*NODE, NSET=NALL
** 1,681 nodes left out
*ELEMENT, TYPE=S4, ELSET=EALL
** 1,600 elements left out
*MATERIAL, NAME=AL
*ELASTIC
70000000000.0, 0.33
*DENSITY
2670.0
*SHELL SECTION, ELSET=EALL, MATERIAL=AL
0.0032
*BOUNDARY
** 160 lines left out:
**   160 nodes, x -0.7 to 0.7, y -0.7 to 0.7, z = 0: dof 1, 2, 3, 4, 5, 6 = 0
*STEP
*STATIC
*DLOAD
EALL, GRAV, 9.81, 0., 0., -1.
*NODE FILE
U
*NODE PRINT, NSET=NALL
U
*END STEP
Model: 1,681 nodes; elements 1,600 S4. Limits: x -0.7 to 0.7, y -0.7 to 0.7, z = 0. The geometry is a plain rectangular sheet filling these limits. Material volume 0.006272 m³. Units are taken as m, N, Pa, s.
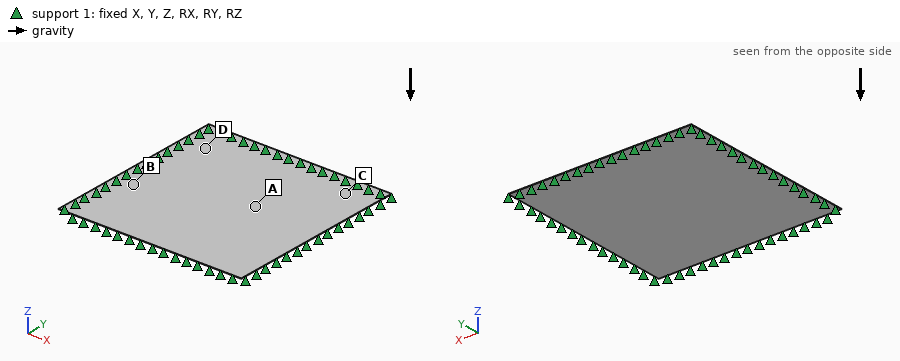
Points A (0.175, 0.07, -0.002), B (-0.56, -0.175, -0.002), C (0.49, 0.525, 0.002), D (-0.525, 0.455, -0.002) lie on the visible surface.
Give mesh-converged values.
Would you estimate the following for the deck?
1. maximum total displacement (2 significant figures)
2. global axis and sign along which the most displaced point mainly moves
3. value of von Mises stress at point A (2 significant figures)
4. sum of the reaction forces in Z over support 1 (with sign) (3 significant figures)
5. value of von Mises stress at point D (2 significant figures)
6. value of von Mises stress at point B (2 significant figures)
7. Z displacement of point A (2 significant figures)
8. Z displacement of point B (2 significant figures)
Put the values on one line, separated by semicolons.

0.0019 m; -Z; 2.0e+06 Pa; 164 N; 1.3e+06 Pa; 1.4e+06 Pa; -0.0016 m; -2.5e-04 m
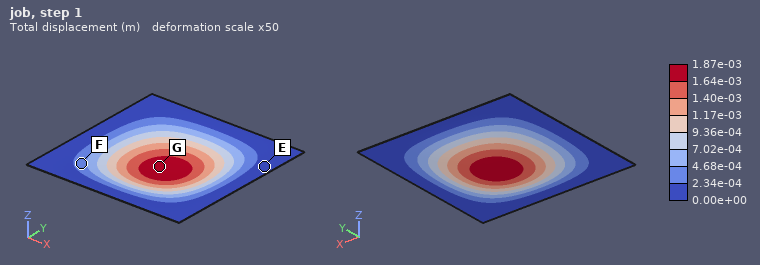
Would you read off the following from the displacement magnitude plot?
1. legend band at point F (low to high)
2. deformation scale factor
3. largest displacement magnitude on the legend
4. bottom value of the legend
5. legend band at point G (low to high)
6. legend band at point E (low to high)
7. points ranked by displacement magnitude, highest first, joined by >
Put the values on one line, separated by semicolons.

2.34e-04 to 4.68e-04 m; 50; 1.87e-03 m; 0.00e+00 m; 1.64e-03 to 1.87e-03 m; 0.00e+00 to 2.34e-04 m; G > F > E
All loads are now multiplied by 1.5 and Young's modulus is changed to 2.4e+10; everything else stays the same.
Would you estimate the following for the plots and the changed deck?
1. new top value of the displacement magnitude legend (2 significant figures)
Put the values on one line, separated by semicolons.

0.0082 m
